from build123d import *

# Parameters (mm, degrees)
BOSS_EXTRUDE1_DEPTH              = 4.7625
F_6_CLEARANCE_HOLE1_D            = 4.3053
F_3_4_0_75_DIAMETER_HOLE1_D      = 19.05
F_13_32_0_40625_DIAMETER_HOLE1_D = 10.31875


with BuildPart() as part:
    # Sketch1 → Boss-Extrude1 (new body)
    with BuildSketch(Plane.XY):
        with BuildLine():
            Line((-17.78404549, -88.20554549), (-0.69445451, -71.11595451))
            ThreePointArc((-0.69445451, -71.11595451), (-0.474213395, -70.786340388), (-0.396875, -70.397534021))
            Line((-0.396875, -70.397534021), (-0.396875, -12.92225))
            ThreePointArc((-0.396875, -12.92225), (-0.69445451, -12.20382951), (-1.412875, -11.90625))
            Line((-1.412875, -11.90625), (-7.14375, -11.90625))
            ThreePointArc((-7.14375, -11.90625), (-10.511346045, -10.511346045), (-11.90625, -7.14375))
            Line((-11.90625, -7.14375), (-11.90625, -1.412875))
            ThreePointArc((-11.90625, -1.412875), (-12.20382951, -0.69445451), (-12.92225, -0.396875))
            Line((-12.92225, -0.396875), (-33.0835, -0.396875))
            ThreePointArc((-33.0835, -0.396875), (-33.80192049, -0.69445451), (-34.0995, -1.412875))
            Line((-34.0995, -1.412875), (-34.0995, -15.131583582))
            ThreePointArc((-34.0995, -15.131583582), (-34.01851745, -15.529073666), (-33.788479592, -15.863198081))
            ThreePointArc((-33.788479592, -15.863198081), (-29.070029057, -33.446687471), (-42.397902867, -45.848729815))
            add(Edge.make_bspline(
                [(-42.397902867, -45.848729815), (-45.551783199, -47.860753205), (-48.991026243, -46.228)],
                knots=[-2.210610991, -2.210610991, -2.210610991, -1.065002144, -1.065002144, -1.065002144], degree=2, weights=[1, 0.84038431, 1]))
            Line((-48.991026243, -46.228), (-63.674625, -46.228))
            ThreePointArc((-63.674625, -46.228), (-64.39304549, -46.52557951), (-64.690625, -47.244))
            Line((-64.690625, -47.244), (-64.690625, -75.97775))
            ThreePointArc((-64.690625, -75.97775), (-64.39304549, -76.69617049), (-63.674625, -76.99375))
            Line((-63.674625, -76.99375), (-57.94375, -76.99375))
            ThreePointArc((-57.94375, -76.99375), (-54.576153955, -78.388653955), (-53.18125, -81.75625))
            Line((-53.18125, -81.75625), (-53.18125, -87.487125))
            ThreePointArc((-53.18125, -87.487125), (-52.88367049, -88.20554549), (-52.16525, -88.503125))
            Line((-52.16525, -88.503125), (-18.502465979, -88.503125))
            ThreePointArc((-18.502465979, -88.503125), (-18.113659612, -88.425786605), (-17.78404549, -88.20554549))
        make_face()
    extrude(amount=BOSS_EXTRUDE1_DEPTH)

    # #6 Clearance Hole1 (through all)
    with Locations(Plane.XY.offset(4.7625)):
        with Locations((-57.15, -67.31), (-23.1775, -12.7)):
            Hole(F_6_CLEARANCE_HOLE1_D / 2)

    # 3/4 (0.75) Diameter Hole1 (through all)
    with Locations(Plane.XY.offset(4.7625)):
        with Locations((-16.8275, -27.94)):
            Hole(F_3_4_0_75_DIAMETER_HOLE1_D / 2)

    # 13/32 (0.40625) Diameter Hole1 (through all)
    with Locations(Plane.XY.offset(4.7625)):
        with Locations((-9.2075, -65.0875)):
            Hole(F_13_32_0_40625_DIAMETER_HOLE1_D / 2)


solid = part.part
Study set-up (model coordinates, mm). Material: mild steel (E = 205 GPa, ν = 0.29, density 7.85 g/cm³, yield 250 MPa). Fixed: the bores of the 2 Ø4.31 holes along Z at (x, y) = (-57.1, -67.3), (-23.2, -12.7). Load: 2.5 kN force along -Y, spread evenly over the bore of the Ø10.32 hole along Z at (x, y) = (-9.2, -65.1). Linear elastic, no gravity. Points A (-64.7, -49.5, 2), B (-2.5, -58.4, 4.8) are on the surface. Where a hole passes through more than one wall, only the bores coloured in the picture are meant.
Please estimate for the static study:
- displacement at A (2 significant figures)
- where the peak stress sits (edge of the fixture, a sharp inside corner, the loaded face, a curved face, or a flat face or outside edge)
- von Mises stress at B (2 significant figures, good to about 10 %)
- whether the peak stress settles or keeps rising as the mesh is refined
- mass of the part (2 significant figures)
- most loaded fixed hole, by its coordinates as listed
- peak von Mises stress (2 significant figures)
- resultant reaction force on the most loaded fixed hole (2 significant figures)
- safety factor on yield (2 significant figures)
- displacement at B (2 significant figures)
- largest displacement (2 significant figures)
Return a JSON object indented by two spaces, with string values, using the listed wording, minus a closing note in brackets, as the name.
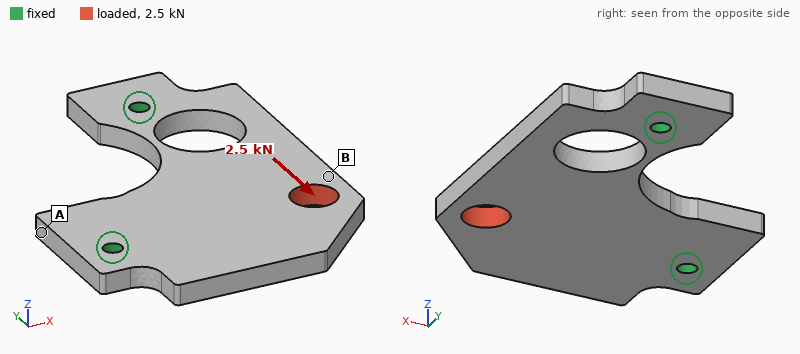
{
  "displacement at A": "4.5 µm",
  "where the peak stress sits": "a curved face",
  "von Mises stress at B": "37 MPa",
  "whether the peak stress settles or keeps rising as the mesh is refined": "settles",
  "mass of the part": "130 g",
  "most loaded fixed hole, by its coordinates as listed": "(-23.2, -12.7)",
  "peak von Mises stress": "190 MPa",
  "resultant reaction force on the most loaded fixed hole": "2.3 kN",
  "safety factor on yield": "1.3",
  "displacement at B": "16 µm",
  "largest displacement": "18 µm"
}
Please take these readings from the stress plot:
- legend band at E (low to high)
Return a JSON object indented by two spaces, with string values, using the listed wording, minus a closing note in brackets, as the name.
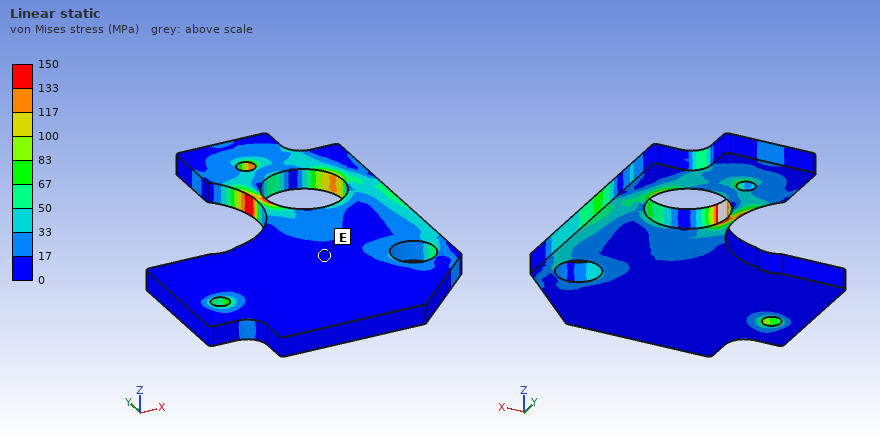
{
  "legend band at E": "0 to 17 MPa"
}
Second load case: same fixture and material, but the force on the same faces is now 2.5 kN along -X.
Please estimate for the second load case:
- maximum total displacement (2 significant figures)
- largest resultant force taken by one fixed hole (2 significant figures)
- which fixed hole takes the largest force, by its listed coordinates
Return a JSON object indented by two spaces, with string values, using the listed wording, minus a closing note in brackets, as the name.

{
  "maximum total displacement": "7.2 µm",
  "largest resultant force taken by one fixed hole": "2.4 kN",
  "which fixed hole takes the largest force, by its listed coordinates": "(-57.1, -67.3)"
}
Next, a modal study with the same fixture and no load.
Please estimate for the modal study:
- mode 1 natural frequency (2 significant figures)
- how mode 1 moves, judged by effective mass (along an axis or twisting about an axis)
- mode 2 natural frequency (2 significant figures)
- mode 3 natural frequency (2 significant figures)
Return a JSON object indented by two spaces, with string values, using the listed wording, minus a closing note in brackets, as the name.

{
  "mode 1 natural frequency": "1600 Hz",
  "how mode 1 moves, judged by effective mass": "along Z",
  "mode 2 natural frequency": "4000 Hz",
  "mode 3 natural frequency": "6500 Hz"
}
